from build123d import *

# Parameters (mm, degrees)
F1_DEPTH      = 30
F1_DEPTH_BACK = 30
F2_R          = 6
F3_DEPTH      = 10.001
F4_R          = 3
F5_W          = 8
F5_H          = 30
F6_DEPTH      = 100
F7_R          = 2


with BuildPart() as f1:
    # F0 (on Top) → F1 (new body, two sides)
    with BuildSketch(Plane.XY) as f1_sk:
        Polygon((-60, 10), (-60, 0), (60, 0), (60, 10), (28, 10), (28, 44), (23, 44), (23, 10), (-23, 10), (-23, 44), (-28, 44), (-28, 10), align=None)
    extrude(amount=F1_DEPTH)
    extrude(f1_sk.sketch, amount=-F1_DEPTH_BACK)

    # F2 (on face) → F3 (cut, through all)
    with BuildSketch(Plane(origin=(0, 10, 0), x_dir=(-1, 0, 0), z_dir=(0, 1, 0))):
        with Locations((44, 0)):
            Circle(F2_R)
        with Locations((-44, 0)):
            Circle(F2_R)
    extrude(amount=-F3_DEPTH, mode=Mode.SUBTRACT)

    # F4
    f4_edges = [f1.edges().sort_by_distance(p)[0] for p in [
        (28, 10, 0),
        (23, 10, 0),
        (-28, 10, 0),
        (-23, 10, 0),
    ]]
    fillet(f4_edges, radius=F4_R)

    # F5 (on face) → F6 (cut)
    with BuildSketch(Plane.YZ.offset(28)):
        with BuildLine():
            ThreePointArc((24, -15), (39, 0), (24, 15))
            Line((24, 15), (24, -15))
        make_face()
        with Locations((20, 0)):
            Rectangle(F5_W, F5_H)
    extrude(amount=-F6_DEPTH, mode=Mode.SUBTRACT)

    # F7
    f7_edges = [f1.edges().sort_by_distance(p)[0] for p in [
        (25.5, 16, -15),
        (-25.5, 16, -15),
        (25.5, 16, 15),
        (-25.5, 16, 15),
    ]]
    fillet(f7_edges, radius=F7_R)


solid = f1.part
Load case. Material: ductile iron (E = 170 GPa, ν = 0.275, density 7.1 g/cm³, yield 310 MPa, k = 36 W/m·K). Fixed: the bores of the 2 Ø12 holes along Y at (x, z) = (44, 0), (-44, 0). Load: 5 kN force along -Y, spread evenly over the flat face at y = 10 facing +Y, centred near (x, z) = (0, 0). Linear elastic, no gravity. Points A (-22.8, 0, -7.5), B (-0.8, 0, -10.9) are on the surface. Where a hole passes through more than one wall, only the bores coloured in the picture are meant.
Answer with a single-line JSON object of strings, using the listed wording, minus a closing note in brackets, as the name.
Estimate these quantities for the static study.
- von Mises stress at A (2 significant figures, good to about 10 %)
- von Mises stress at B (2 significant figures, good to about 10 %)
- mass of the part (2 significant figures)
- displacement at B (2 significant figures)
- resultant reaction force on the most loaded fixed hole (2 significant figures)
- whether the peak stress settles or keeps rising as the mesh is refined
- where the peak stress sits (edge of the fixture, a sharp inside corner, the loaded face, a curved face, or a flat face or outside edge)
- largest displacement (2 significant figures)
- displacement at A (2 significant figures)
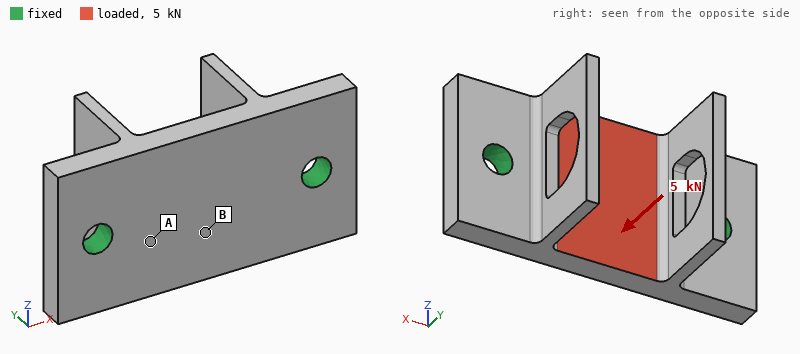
{"von Mises stress at A": "8.6 MPa", "von Mises stress at B": "31 MPa", "mass of the part": "600 g", "displacement at B": "20 µm", "resultant reaction force on the most loaded fixed hole": "2.5 kN", "whether the peak stress settles or keeps rising as the mesh is refined": "keeps rising", "where the peak stress sits": "edge of the fixture", "largest displacement": "28 µm", "displacement at A": "11 µm"}
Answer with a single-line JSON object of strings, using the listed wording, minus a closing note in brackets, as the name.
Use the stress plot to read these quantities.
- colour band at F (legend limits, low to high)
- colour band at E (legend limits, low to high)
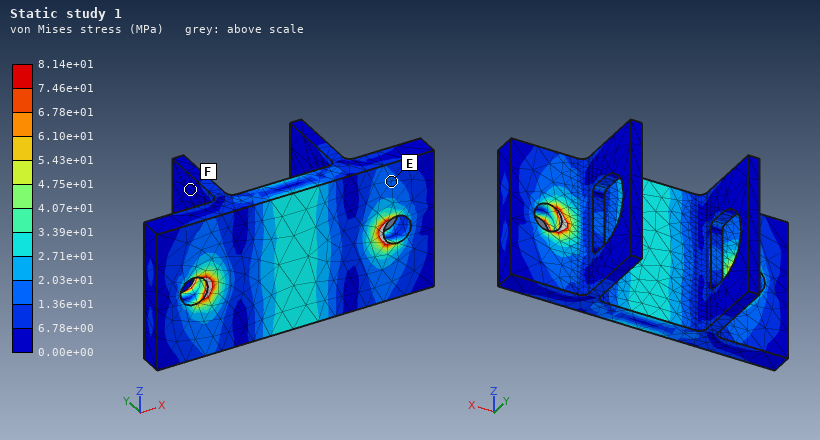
{"colour band at F": "0.00e+00 to 6.78e+00 MPa", "colour band at E": "1.36e+01 to 2.03e+01 MPa"}
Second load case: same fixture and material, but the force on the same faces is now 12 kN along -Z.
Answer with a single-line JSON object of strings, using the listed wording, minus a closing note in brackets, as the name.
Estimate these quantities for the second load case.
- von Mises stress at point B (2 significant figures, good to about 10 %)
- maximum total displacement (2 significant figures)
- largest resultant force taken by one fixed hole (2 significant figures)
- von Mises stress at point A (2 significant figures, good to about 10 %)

{"von Mises stress at point B": "13 MPa", "maximum total displacement": "25 µm", "largest resultant force taken by one fixed hole": "6.0 kN", "von Mises stress at point A": "9.5 MPa"}
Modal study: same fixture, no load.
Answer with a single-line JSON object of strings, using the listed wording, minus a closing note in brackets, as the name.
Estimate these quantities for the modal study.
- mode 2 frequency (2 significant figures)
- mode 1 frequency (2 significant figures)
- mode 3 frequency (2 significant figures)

{"mode 2 frequency": "2700 Hz", "mode 1 frequency": "2600 Hz", "mode 3 frequency": "3900 Hz"}
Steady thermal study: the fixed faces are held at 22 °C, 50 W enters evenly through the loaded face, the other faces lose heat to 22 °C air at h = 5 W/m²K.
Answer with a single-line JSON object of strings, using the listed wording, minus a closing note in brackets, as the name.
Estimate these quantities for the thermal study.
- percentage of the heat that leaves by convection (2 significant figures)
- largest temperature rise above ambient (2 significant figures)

{"percentage of the heat that leaves by convection": "4.5 %", "largest temperature rise above ambient": "43 K"}
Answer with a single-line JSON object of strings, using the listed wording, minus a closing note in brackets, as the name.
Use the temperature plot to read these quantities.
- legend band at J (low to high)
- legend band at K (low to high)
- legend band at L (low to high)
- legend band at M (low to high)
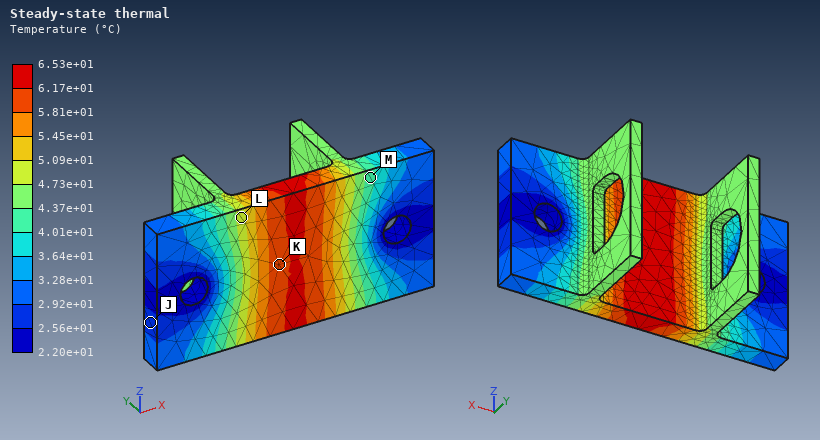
{"legend band at J": "2.56e+01 to 2.92e+01 °C", "legend band at K": "5.81e+01 to 6.17e+01 °C", "legend band at L": "4.73e+01 to 5.09e+01 °C", "legend band at M": "4.01e+01 to 4.37e+01 °C"}
